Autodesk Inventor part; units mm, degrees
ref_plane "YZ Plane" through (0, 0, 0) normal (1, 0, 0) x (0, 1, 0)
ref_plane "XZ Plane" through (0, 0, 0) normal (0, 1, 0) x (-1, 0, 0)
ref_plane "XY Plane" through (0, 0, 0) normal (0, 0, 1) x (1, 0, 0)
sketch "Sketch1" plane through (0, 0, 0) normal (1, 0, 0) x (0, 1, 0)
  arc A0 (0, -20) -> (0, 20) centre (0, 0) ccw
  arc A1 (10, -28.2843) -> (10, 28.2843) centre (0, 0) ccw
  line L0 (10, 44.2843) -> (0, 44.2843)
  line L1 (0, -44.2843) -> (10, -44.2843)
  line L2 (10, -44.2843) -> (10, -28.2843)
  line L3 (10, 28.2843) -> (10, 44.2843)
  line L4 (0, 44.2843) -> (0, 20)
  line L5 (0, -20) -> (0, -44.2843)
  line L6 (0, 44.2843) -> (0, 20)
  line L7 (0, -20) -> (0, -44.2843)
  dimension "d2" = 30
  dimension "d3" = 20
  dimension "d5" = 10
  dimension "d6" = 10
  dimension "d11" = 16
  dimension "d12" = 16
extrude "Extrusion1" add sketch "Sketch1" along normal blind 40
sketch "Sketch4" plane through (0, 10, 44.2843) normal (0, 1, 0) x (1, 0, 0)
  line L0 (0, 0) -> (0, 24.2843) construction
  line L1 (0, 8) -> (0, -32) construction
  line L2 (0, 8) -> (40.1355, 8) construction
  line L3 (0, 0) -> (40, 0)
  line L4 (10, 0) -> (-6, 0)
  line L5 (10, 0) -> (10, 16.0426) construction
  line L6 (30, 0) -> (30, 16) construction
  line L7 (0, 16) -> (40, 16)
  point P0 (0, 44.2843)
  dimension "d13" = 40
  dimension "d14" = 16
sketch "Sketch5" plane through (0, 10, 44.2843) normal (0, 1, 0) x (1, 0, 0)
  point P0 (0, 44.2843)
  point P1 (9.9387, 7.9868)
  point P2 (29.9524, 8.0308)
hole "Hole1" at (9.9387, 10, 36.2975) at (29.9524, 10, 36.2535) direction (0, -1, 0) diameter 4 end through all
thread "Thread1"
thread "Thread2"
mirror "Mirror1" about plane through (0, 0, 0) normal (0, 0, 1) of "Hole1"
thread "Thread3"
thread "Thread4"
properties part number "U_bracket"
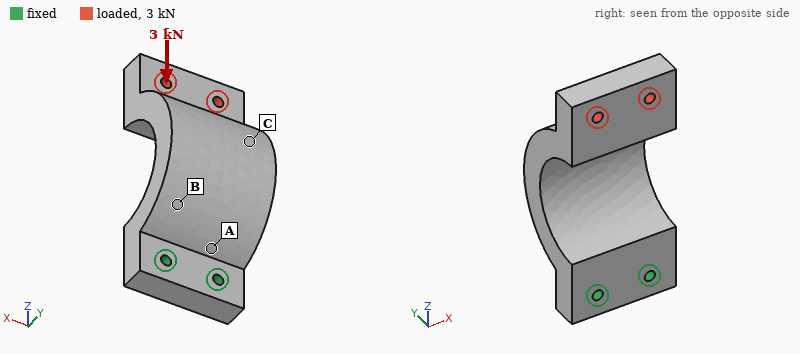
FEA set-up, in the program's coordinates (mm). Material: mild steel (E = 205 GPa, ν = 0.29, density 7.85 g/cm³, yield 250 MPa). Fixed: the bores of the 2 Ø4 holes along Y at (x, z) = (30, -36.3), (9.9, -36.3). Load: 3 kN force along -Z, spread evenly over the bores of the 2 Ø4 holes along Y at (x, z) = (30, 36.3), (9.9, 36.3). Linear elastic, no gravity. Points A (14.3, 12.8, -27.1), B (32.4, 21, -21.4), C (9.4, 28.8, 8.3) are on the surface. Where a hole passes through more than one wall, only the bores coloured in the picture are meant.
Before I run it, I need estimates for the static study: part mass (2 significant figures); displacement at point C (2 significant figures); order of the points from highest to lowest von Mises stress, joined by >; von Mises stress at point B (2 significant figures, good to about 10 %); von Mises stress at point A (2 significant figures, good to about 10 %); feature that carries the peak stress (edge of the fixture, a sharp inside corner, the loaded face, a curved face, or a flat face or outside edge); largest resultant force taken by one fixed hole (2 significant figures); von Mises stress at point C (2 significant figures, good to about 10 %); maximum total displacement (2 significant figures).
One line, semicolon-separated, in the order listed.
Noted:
340 g; 0.043 mm; C > B > A; 43 MPa; 18 MPa; a curved face; 1.5 kN; 63 MPa; 0.19 mm
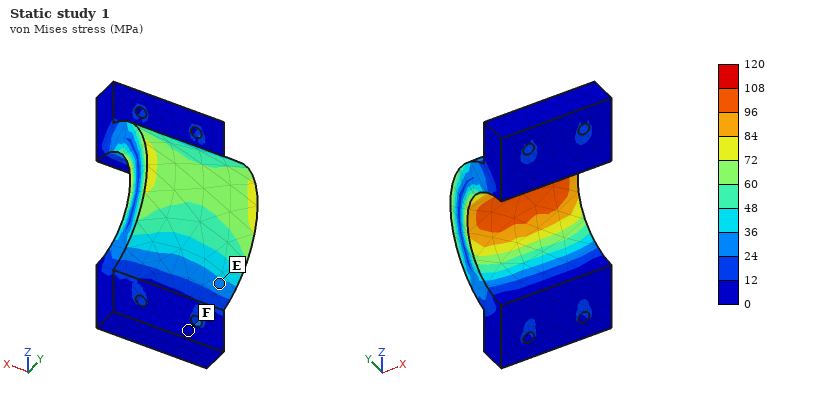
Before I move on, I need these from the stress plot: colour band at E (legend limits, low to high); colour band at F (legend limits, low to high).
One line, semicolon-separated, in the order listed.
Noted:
24 to 36 MPa; 0 to 12 MPa
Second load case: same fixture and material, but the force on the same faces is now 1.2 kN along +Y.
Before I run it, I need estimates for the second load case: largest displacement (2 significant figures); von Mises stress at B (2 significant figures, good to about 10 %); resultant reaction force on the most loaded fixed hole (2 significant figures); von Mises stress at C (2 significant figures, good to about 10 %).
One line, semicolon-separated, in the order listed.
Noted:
0.34 mm; 80 MPa; 640 N; 44 MPa
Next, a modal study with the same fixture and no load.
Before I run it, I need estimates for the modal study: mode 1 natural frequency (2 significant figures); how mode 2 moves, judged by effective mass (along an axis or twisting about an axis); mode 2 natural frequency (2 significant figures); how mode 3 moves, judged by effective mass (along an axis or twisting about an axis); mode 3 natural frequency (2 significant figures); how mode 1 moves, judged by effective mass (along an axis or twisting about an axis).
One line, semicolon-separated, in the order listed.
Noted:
1000 Hz; along X; 1900 Hz; along Z; 3500 Hz; along Y
